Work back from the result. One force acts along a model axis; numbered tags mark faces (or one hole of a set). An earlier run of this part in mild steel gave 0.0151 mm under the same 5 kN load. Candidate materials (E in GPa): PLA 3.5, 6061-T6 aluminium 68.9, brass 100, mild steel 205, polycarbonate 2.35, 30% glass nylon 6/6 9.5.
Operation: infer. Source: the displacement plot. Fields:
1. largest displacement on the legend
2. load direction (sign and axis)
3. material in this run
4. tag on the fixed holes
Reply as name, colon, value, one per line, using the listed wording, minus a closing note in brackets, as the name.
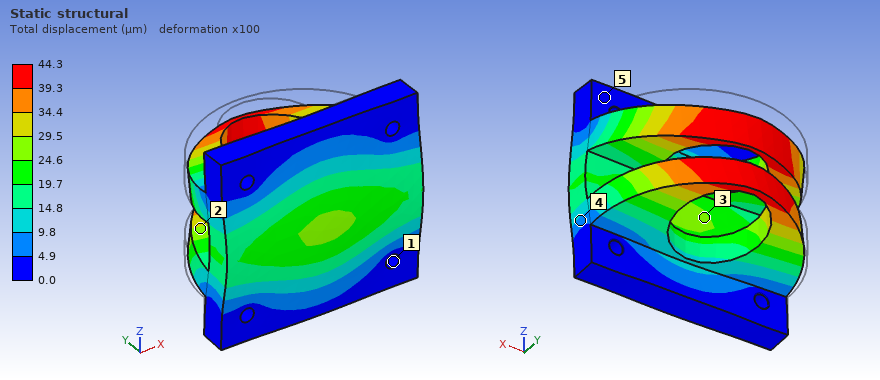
largest displacement on the legend: 44.3 µm
load direction: -Y
material in this run: 6061-T6 aluminium
tag on the fixed holes: 1
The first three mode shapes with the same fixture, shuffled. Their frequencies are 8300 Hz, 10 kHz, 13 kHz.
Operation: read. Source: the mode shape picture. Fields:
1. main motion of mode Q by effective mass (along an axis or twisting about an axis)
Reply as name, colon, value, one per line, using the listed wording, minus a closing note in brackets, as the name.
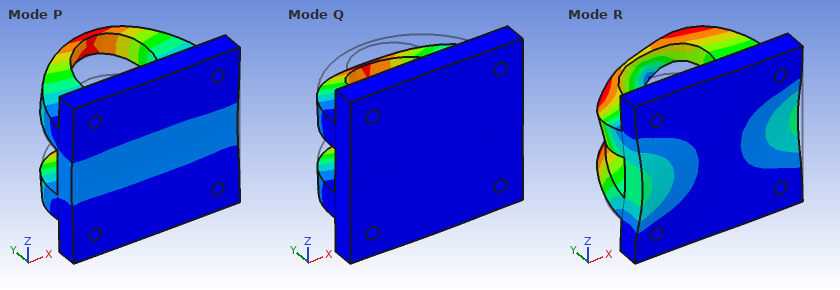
main motion of mode Q by effective mass: along Z
